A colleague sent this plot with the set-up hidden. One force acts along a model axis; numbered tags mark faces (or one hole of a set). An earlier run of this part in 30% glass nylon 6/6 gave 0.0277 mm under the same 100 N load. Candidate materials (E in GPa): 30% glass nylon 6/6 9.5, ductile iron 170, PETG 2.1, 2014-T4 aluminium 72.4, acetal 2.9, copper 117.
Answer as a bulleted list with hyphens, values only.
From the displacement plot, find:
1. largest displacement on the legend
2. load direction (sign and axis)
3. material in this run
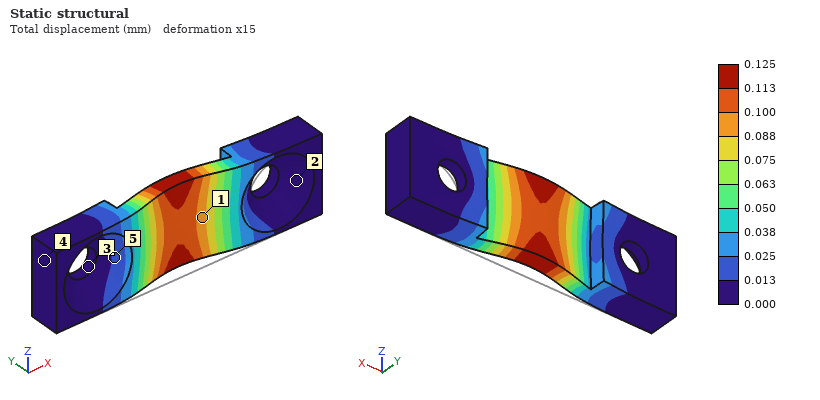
- 0.125 mm
- +Y
- PETG
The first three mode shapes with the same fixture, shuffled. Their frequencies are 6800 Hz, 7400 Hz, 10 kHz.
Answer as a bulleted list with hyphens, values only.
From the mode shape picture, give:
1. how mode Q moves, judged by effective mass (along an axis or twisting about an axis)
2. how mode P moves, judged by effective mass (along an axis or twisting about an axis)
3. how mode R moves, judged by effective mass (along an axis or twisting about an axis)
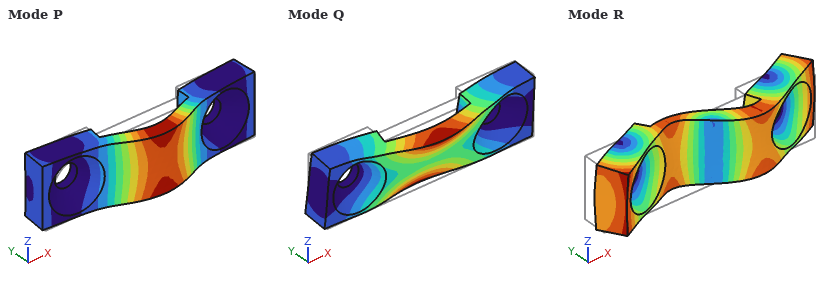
- along Z
- along Y
- along X
